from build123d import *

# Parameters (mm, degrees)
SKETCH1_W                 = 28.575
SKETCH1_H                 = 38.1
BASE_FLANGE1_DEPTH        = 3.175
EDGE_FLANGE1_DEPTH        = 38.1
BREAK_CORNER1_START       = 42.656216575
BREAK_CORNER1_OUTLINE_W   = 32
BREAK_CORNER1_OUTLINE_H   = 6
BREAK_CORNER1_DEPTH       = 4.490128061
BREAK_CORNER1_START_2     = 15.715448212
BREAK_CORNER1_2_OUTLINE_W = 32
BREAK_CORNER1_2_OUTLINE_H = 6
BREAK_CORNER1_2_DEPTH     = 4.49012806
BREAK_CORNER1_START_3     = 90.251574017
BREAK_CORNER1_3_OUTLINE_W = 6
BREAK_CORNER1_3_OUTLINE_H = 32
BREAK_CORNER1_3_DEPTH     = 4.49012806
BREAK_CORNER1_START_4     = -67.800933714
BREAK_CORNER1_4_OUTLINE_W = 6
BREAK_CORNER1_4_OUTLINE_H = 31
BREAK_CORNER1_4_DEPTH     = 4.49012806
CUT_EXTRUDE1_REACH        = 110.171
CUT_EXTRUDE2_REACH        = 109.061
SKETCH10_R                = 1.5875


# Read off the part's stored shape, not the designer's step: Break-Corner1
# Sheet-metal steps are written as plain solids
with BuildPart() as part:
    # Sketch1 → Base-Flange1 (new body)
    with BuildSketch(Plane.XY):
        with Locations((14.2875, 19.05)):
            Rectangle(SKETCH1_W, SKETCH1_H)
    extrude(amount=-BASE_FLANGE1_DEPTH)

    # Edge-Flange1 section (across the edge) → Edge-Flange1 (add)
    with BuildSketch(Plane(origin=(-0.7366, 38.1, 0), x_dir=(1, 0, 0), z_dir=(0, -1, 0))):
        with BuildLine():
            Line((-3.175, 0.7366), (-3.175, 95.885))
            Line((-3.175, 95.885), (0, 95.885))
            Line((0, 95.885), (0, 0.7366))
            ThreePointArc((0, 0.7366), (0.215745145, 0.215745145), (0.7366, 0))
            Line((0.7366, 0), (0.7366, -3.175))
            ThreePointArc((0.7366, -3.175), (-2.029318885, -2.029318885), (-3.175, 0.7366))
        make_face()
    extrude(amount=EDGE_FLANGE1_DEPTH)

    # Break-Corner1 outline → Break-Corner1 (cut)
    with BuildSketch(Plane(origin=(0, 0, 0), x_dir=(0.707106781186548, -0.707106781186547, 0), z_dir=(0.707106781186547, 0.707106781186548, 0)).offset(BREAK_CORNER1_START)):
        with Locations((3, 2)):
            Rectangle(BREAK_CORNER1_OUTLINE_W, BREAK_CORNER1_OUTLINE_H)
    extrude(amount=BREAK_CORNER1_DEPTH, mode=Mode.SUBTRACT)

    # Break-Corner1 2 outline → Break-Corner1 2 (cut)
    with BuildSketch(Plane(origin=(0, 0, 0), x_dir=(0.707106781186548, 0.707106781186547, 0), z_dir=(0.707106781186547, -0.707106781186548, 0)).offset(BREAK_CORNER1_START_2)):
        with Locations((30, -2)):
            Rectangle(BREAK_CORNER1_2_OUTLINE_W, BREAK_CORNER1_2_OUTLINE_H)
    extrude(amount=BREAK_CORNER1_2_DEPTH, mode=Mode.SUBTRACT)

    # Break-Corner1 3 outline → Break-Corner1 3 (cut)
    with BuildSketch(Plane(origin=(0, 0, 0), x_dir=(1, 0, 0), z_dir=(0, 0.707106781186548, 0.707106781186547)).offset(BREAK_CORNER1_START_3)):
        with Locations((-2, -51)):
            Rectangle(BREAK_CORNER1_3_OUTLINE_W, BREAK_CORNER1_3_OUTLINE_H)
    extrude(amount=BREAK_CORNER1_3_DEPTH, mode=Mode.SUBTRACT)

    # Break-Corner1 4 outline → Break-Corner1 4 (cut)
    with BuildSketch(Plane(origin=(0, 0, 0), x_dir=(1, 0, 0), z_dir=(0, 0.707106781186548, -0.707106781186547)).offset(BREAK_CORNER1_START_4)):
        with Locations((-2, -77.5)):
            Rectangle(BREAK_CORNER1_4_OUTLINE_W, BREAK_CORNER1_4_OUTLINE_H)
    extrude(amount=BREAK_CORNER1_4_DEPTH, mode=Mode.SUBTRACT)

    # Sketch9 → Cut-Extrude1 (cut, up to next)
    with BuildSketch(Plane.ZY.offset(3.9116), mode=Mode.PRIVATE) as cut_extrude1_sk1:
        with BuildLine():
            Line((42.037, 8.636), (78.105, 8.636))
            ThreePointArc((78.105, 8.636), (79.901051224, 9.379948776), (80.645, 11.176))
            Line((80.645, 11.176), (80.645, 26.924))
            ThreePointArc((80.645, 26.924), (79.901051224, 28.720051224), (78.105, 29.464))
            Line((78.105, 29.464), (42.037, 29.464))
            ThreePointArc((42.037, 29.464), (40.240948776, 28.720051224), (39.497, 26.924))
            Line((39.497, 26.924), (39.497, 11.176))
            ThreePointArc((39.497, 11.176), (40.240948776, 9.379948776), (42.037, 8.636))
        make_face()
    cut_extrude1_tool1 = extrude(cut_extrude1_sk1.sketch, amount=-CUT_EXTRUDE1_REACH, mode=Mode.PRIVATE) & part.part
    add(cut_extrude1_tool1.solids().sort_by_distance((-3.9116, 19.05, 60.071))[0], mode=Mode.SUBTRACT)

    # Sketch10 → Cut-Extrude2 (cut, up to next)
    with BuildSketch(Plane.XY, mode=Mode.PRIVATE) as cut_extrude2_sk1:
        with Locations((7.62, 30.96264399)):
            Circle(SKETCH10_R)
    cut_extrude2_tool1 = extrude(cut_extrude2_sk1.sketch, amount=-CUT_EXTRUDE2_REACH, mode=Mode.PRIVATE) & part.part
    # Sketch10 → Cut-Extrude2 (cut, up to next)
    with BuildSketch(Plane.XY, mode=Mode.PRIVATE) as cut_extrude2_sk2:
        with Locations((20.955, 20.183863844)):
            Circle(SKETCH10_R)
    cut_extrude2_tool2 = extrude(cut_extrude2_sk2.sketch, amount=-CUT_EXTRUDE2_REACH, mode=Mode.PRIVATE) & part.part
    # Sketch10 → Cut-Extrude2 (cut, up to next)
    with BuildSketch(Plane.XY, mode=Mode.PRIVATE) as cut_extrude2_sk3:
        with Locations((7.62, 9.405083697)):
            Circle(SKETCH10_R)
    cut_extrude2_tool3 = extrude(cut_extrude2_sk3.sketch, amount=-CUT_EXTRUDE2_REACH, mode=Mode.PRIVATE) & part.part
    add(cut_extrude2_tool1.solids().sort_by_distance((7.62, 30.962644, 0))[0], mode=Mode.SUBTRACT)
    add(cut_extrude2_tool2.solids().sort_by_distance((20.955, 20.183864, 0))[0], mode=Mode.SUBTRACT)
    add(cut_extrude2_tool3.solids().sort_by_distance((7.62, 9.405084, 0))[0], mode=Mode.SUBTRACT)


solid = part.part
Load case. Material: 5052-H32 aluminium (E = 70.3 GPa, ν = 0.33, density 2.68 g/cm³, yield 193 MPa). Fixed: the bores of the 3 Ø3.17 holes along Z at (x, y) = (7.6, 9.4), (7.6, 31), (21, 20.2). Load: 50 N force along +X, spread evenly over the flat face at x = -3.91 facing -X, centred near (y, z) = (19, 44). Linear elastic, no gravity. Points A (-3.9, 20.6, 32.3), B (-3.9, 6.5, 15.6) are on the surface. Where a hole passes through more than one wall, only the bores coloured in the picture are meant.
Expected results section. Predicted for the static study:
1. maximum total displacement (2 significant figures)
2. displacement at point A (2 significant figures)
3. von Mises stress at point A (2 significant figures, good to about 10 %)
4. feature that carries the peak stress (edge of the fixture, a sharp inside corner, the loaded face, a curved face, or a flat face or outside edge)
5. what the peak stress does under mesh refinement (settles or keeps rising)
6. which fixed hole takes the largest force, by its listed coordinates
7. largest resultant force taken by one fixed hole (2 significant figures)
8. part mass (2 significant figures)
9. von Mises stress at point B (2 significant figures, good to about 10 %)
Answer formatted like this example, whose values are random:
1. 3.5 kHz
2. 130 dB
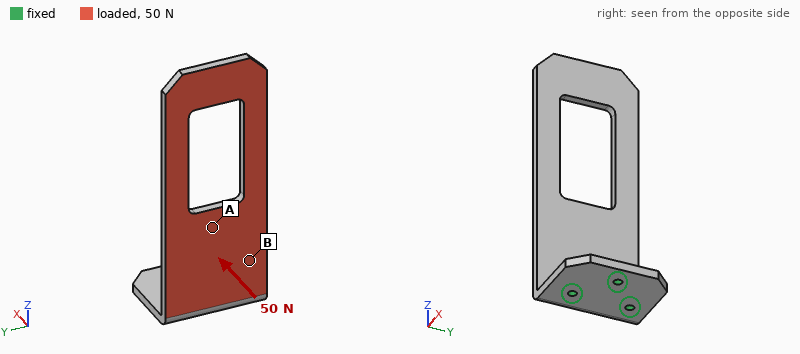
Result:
1. 1.1 mm
2. 0.23 mm
3. 9.8 MPa
4. edge of the fixture
5. keeps rising
6. (21, 20.2)
7. 44 N
8. 33 g
9. 23 MPa
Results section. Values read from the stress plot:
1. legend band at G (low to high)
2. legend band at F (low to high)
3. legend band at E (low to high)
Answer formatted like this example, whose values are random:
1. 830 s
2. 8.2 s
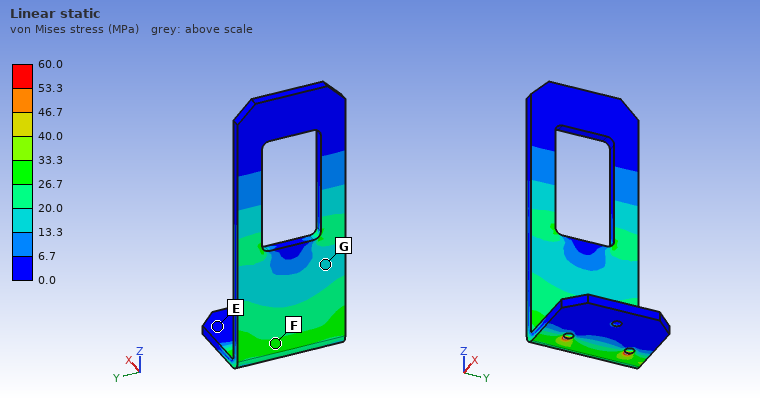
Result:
1. 13.3 to 20.0 MPa
2. 26.7 to 33.3 MPa
3. 0.0 to 6.7 MPa
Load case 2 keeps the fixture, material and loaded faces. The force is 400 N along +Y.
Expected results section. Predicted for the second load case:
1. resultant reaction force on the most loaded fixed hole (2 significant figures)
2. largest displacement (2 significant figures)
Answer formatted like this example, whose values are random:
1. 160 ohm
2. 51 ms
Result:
1. 820 N
2. 0.48 mm
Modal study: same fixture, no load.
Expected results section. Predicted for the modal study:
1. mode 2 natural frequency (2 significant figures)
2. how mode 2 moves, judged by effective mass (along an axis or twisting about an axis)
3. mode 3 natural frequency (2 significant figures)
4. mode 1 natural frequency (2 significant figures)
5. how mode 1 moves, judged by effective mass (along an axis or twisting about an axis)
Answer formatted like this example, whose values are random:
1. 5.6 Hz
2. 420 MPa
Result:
1. 1100 Hz
2. along Y
3. 1300 Hz
4. 270 Hz
5. along X
